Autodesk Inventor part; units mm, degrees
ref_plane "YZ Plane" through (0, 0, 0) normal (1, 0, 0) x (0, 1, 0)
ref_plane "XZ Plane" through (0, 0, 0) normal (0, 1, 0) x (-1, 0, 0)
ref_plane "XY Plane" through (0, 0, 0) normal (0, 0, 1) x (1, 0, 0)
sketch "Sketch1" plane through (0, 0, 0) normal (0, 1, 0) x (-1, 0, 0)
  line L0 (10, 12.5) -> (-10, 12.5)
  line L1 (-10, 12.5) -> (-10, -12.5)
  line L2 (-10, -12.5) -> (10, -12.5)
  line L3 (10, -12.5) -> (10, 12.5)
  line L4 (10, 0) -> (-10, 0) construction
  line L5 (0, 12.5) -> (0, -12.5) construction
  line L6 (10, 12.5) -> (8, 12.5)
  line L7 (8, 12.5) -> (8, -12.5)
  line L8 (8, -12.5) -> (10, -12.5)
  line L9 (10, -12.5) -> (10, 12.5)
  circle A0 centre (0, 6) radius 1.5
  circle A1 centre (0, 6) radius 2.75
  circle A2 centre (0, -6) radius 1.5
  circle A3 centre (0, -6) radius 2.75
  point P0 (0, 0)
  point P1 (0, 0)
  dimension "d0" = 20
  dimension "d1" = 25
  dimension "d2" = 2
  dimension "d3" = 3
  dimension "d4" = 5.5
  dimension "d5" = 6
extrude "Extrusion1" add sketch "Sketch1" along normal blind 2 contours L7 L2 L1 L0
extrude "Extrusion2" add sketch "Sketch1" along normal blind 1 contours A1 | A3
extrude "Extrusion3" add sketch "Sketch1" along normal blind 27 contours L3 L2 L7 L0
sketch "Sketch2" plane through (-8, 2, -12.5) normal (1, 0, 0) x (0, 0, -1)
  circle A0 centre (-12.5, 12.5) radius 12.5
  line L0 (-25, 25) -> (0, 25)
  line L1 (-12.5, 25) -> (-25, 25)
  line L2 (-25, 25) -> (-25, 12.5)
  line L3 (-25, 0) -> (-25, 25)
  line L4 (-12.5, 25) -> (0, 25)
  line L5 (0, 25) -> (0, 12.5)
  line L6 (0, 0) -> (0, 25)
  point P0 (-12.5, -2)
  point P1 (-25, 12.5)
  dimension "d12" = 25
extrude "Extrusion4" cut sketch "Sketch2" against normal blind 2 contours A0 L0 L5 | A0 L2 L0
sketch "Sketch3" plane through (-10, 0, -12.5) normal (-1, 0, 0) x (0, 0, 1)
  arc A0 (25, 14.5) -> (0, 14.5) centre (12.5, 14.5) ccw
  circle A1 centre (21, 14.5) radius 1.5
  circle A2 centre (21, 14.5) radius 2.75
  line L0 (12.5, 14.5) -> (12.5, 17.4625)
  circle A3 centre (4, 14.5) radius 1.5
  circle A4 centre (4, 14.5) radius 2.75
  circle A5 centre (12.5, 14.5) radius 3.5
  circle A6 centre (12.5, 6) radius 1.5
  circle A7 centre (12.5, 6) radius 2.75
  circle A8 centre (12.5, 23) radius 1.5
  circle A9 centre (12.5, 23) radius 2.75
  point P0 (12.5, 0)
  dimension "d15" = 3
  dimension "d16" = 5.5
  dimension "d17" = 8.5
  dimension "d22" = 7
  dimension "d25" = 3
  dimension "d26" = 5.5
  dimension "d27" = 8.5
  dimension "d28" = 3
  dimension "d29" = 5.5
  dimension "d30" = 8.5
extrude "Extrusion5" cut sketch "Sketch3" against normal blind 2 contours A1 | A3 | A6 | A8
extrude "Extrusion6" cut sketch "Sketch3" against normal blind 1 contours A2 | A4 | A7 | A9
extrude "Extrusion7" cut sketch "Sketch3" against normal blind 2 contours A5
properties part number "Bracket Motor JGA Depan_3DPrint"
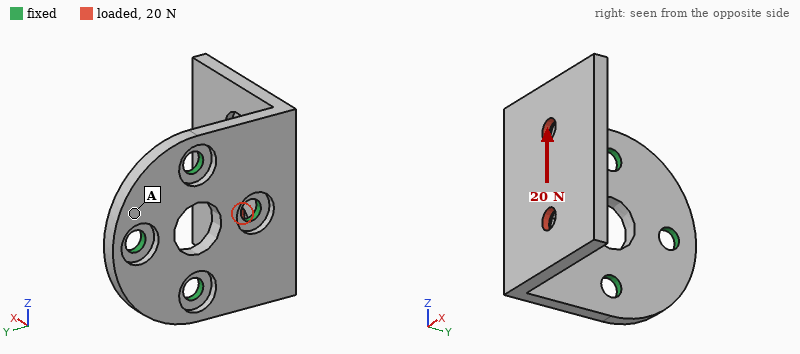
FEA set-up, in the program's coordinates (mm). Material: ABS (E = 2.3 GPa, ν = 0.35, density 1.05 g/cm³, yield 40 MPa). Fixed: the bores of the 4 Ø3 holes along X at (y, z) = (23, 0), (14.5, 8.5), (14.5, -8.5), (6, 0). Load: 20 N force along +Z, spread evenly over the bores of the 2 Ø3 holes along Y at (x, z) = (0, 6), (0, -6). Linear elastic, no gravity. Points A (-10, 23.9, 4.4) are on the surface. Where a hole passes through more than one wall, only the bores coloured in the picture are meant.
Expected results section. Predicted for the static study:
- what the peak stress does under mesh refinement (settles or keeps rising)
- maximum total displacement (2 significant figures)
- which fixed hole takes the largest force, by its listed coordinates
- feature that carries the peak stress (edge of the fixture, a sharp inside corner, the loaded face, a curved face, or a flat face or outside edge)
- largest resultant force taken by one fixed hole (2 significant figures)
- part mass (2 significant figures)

keeps rising
0.42 mm
(6, 0)
edge of the fixture
28 N
1.9 g
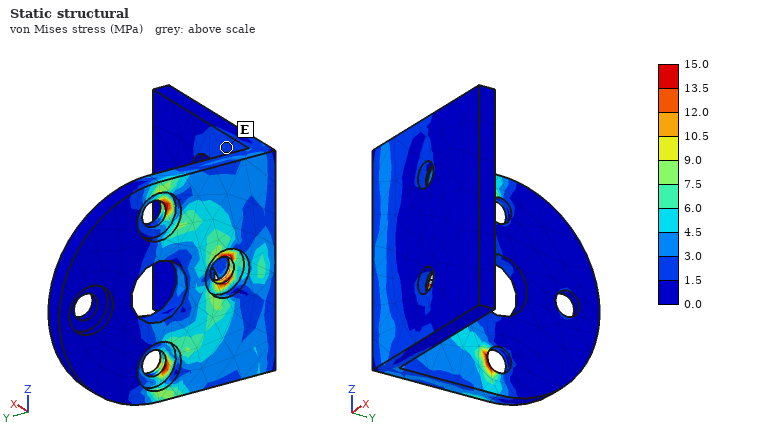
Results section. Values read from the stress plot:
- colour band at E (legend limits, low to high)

1.5 to 3.0 MPa
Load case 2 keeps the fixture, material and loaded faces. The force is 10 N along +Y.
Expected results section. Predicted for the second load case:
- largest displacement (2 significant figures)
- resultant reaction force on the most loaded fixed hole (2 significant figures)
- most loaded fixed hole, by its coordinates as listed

0.44 mm
16 N
(6, 0)
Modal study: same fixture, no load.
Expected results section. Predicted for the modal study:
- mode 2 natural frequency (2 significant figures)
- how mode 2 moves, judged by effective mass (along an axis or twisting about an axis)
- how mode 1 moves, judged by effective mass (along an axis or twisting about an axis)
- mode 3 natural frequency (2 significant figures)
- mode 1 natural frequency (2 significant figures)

1200 Hz
along Z
along Y
2300 Hz
870 Hz
